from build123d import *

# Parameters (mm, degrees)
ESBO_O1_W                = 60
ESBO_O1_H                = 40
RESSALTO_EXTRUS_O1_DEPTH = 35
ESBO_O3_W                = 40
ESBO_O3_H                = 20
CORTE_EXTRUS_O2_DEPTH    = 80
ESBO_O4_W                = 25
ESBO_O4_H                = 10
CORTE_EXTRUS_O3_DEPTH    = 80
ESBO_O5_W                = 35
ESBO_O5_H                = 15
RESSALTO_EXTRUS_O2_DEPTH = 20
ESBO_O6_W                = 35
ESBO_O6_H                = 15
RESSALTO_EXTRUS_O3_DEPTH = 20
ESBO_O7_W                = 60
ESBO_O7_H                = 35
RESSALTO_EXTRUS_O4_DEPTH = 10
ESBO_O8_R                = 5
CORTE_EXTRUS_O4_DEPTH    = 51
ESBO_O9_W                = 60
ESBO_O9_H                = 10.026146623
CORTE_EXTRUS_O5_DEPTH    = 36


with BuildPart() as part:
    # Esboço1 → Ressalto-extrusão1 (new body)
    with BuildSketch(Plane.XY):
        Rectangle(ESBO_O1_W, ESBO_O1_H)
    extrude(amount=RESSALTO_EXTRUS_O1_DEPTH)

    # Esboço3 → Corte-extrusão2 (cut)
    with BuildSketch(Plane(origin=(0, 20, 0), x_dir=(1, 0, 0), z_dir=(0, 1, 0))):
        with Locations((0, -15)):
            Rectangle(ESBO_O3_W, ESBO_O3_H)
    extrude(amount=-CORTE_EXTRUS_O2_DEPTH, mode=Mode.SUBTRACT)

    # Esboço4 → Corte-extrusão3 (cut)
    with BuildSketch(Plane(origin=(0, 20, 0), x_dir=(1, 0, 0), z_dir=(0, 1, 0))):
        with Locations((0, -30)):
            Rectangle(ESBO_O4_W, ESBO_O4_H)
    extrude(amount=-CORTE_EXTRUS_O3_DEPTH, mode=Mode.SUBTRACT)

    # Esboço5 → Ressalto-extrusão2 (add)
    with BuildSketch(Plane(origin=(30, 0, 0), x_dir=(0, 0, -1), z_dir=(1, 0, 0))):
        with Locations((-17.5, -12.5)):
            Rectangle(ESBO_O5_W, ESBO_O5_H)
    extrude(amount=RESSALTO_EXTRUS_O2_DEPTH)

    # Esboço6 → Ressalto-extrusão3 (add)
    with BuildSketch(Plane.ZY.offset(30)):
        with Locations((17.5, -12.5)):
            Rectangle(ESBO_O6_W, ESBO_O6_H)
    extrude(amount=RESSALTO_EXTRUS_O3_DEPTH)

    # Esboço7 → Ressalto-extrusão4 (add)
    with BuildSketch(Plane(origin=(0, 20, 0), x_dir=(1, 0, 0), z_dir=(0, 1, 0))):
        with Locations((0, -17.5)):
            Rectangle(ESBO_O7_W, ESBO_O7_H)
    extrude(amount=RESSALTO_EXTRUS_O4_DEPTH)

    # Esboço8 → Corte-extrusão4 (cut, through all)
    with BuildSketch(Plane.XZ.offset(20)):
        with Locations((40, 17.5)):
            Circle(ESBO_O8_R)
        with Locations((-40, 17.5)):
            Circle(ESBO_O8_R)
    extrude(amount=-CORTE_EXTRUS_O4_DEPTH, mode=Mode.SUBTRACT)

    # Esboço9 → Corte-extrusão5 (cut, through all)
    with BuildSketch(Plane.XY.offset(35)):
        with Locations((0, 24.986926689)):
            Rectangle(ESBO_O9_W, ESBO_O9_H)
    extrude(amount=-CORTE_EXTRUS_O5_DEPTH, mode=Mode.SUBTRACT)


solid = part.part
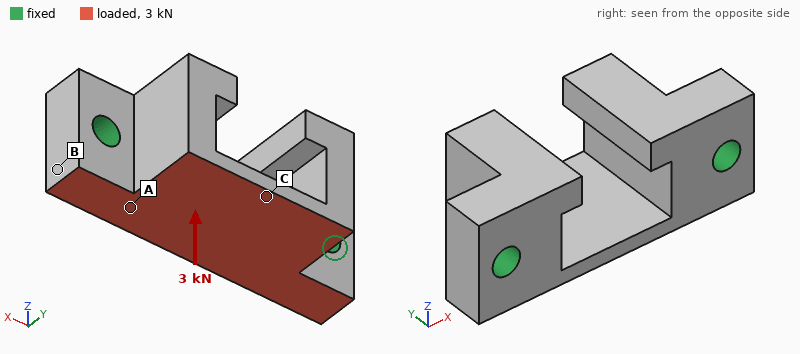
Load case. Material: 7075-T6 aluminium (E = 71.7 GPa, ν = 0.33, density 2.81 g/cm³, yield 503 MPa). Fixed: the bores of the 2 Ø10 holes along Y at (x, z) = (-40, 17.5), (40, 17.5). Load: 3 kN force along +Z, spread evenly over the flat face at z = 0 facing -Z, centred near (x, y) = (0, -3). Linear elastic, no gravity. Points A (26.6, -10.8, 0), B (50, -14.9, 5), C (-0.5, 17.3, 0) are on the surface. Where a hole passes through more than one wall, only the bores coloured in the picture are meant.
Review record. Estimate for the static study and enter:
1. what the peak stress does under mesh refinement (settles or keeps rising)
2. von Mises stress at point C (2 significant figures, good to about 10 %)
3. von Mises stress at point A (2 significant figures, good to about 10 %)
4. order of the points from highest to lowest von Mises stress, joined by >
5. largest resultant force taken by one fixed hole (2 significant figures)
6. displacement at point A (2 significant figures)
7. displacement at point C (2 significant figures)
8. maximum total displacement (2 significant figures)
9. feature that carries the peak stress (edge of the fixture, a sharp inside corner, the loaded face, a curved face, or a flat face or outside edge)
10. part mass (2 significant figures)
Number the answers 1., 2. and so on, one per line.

1. keeps rising
2. 22 MPa
3. 7.7 MPa
4. C > A > B
5. 1.7 kN
6. 5.4 µm
7. 32 µm
8. 34 µm
9. edge of the fixture
10. 170 g
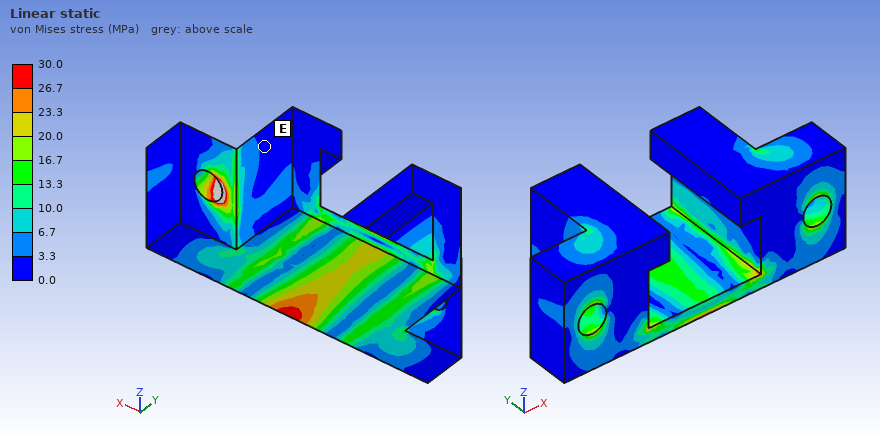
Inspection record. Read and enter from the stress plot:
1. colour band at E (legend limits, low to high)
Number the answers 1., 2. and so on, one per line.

1. 0.0 to 3.3 MPa
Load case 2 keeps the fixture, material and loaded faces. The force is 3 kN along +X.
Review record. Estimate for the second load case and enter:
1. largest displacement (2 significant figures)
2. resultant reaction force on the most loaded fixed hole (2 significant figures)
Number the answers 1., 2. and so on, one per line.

1. 9.6 µm
2. 1.6 kN
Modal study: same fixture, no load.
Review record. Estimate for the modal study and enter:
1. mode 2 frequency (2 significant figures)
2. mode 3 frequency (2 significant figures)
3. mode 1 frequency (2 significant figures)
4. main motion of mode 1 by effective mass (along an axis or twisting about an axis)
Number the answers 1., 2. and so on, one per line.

1. 7300 Hz
2. 8000 Hz
3. 6800 Hz
4. along Z
